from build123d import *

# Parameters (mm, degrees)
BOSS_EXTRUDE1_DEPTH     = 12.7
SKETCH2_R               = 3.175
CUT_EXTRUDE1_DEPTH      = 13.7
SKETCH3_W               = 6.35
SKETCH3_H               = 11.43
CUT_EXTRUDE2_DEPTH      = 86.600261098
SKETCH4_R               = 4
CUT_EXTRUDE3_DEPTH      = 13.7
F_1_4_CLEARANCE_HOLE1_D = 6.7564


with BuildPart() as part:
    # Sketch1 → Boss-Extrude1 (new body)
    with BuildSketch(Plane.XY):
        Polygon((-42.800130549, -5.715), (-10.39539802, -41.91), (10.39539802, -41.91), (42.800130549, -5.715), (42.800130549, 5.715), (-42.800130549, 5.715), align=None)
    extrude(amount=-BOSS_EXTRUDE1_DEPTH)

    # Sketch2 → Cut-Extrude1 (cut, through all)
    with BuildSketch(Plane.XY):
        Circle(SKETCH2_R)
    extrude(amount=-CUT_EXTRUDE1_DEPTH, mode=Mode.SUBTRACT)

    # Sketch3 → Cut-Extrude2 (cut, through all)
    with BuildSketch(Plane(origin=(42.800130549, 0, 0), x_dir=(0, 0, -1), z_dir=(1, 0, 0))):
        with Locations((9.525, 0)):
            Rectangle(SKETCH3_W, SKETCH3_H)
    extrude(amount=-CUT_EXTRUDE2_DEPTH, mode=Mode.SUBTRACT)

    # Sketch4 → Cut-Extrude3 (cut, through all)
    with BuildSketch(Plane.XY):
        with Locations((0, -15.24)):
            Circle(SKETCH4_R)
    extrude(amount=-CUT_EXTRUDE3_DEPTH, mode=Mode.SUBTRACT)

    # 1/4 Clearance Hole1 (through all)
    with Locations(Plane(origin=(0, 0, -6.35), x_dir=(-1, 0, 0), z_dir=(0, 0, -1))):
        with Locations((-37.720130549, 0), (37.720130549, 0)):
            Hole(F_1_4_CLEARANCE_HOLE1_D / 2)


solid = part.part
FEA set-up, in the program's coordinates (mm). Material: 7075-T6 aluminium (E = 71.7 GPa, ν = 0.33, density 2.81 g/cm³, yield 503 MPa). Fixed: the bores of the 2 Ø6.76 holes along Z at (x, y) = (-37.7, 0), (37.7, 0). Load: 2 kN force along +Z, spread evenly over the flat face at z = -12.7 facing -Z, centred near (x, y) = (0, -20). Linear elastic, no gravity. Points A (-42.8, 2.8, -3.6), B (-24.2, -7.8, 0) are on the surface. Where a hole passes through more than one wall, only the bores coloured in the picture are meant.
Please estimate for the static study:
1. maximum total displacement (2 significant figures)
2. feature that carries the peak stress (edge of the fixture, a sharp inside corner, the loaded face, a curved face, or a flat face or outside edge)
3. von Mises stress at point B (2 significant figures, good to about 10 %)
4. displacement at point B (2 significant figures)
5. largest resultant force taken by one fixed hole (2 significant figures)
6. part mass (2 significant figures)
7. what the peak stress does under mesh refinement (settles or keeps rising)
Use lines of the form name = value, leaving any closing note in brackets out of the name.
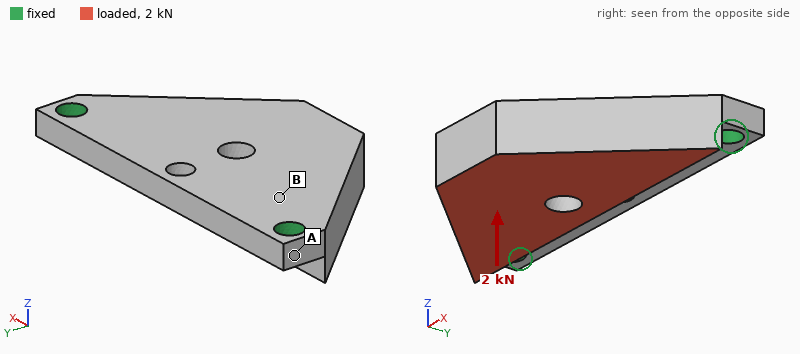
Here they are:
maximum total displacement = 0.23 mm
feature that carries the peak stress = edge of the fixture
von Mises stress at point B = 37 MPa
displacement at point B = 0.035 mm
largest resultant force taken by one fixed hole = 1.1 kN
part mass = 83 g
what the peak stress does under mesh refinement = keeps rising
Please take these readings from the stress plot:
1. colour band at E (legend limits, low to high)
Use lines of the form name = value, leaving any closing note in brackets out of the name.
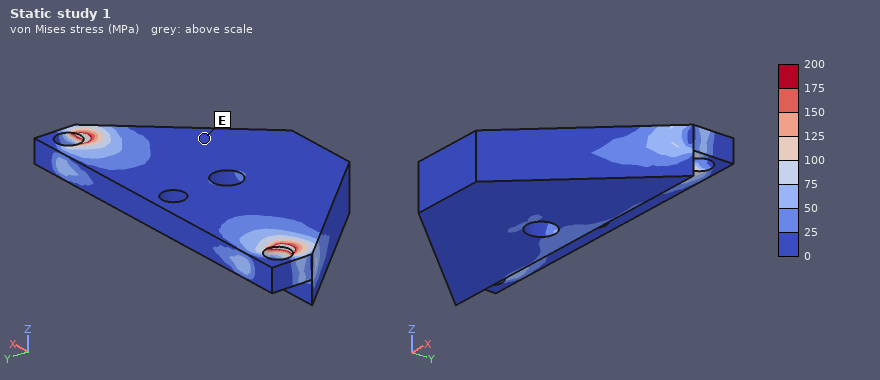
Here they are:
colour band at E = 0 to 25 MPa
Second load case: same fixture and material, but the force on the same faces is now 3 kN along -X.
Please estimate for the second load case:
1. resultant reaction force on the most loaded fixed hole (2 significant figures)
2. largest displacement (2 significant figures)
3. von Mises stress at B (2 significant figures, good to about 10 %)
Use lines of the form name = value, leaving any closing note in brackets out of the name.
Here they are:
resultant reaction force on the most loaded fixed hole = 1.7 kN
largest displacement = 8.5 µm
von Mises stress at B = 7.0 MPa
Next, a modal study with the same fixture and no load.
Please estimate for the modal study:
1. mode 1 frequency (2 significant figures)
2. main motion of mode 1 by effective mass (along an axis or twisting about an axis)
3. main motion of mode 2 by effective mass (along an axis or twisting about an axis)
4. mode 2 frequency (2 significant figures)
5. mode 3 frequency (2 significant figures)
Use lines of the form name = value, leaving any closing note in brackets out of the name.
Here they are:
mode 1 frequency = 2300 Hz
main motion of mode 1 by effective mass = along Z
main motion of mode 2 by effective mass = along Z
mode 2 frequency = 8300 Hz
mode 3 frequency = 11 kHz
